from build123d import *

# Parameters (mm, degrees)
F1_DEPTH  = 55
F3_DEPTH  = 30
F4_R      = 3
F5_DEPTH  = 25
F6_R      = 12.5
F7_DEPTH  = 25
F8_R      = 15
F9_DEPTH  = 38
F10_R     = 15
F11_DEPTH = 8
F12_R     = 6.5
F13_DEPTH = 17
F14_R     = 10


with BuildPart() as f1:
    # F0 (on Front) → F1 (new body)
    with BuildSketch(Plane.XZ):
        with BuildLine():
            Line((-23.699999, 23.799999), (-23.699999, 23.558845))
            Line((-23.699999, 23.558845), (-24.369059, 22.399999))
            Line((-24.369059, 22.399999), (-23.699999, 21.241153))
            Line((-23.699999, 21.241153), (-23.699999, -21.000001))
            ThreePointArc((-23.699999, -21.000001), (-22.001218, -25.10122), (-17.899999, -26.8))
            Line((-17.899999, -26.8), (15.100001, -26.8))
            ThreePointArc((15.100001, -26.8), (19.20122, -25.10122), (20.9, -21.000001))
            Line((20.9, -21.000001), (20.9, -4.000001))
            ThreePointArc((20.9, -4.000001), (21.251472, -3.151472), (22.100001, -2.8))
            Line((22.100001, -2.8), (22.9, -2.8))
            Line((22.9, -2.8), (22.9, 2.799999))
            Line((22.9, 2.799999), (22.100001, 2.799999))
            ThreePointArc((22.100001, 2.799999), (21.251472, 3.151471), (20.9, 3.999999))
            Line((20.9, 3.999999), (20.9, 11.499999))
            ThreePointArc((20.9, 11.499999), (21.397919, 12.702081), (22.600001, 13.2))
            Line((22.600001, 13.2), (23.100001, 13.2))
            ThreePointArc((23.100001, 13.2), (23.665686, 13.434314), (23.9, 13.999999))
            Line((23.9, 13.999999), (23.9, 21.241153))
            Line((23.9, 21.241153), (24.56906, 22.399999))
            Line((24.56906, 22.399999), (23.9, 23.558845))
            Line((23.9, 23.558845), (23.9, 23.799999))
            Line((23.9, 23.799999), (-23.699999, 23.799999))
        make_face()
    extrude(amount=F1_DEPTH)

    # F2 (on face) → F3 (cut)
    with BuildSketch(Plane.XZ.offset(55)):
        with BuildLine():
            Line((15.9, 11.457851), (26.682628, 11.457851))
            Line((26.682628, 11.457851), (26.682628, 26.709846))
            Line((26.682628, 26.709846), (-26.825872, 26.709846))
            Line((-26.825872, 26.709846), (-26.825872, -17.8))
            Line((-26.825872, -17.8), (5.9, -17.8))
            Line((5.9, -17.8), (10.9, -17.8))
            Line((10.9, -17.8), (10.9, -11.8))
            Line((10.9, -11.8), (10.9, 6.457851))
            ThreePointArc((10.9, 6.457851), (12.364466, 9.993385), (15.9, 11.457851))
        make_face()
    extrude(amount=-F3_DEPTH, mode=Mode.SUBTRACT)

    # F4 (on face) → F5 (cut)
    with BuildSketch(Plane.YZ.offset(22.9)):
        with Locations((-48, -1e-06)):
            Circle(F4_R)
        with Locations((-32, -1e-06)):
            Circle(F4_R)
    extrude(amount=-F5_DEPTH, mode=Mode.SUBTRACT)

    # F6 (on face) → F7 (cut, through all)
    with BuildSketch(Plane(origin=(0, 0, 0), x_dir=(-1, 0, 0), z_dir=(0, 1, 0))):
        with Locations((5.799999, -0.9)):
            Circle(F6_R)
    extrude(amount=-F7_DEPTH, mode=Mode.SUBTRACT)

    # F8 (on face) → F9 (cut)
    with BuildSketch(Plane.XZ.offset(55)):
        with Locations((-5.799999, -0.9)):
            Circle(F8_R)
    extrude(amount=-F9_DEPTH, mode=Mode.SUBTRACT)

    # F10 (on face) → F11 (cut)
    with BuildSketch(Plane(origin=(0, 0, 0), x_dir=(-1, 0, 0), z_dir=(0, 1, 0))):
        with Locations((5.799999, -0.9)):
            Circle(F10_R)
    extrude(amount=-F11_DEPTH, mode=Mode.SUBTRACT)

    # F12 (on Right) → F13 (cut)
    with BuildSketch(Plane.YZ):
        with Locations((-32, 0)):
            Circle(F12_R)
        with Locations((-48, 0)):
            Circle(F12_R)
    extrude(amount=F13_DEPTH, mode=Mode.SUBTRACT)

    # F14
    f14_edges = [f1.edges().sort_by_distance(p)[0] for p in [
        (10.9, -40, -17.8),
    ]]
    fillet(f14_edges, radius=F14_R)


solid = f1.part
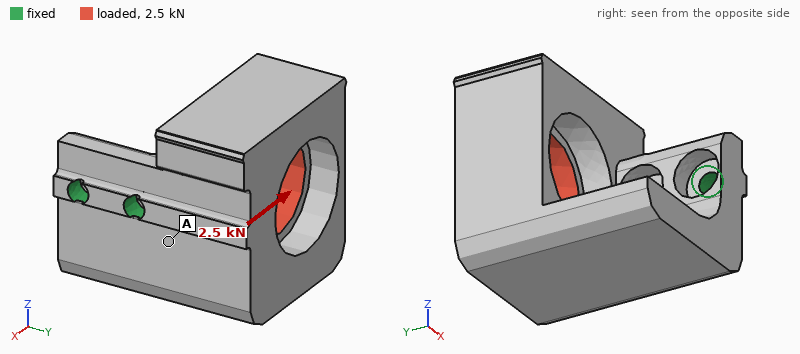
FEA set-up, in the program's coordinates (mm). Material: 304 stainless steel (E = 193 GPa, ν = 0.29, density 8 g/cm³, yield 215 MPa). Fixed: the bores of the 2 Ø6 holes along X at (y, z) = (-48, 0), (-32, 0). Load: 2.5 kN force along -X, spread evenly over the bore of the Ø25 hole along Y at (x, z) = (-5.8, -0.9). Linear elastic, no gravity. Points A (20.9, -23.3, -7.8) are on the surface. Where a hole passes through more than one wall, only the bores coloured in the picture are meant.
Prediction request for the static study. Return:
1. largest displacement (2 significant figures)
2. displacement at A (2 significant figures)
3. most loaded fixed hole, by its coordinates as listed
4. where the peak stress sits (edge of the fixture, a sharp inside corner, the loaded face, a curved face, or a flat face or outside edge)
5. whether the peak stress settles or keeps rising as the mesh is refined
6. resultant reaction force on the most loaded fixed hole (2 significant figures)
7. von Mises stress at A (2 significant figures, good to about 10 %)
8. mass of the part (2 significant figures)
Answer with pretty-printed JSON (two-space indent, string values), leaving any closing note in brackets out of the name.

{
  "largest displacement": "51 µm",
  "displacement at A": "11 µm",
  "most loaded fixed hole, by its coordinates as listed": "(-32, 0)",
  "where the peak stress sits": "edge of the fixture",
  "whether the peak stress settles or keeps rising as the mesh is refined": "keeps rising",
  "resultant reaction force on the most loaded fixed hole": "4.3 kN",
  "von Mises stress at A": "18 MPa",
  "mass of the part": "490 g"
}
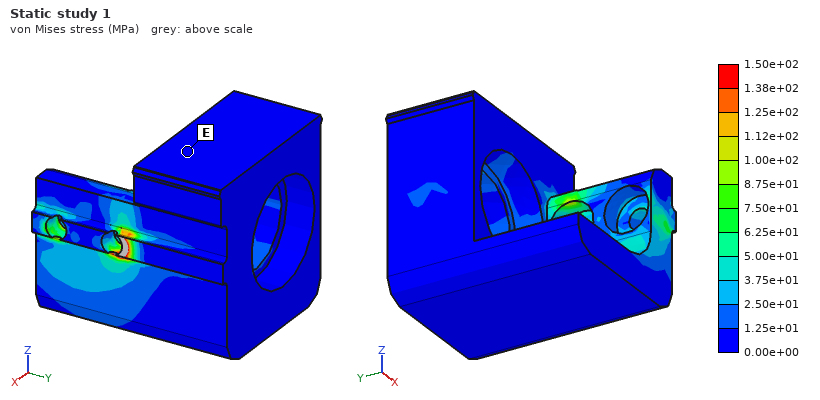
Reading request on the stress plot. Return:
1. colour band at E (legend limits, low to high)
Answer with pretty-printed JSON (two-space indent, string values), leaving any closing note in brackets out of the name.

{
  "colour band at E": "0.00e+00 to 1.25e+01 MPa"
}
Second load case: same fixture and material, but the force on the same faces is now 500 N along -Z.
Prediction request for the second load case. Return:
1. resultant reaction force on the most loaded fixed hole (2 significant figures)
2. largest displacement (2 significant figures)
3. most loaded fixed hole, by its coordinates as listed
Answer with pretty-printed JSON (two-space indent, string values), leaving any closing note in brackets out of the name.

{
  "resultant reaction force on the most loaded fixed hole": "870 N",
  "largest displacement": "29 µm",
  "most loaded fixed hole, by its coordinates as listed": "(-32, 0)"
}
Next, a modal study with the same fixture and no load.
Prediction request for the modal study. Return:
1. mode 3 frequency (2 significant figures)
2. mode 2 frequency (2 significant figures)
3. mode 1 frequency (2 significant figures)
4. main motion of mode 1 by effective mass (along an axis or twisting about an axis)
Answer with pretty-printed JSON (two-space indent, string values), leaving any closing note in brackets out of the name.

{
  "mode 3 frequency": "3800 Hz",
  "mode 2 frequency": "2000 Hz",
  "mode 1 frequency": "1300 Hz",
  "main motion of mode 1 by effective mass": "along Z"
}
